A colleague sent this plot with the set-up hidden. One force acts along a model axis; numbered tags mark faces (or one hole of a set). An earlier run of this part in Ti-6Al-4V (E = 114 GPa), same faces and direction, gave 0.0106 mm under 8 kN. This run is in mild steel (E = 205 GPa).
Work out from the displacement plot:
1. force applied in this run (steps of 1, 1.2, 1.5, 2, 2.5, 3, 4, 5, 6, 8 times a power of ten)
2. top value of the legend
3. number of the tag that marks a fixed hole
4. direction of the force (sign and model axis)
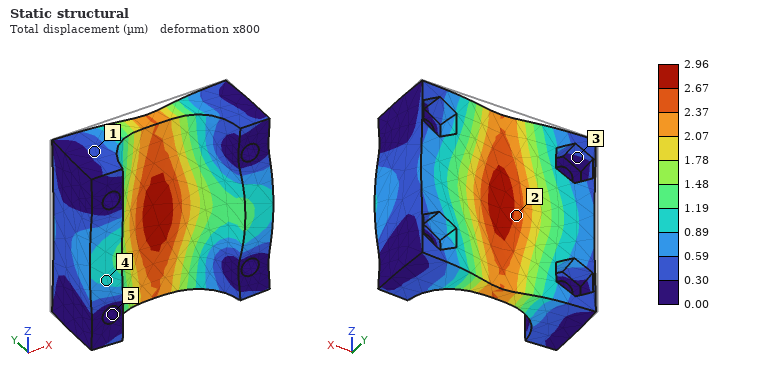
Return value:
4 kN
2.96 µm
5
-Y
